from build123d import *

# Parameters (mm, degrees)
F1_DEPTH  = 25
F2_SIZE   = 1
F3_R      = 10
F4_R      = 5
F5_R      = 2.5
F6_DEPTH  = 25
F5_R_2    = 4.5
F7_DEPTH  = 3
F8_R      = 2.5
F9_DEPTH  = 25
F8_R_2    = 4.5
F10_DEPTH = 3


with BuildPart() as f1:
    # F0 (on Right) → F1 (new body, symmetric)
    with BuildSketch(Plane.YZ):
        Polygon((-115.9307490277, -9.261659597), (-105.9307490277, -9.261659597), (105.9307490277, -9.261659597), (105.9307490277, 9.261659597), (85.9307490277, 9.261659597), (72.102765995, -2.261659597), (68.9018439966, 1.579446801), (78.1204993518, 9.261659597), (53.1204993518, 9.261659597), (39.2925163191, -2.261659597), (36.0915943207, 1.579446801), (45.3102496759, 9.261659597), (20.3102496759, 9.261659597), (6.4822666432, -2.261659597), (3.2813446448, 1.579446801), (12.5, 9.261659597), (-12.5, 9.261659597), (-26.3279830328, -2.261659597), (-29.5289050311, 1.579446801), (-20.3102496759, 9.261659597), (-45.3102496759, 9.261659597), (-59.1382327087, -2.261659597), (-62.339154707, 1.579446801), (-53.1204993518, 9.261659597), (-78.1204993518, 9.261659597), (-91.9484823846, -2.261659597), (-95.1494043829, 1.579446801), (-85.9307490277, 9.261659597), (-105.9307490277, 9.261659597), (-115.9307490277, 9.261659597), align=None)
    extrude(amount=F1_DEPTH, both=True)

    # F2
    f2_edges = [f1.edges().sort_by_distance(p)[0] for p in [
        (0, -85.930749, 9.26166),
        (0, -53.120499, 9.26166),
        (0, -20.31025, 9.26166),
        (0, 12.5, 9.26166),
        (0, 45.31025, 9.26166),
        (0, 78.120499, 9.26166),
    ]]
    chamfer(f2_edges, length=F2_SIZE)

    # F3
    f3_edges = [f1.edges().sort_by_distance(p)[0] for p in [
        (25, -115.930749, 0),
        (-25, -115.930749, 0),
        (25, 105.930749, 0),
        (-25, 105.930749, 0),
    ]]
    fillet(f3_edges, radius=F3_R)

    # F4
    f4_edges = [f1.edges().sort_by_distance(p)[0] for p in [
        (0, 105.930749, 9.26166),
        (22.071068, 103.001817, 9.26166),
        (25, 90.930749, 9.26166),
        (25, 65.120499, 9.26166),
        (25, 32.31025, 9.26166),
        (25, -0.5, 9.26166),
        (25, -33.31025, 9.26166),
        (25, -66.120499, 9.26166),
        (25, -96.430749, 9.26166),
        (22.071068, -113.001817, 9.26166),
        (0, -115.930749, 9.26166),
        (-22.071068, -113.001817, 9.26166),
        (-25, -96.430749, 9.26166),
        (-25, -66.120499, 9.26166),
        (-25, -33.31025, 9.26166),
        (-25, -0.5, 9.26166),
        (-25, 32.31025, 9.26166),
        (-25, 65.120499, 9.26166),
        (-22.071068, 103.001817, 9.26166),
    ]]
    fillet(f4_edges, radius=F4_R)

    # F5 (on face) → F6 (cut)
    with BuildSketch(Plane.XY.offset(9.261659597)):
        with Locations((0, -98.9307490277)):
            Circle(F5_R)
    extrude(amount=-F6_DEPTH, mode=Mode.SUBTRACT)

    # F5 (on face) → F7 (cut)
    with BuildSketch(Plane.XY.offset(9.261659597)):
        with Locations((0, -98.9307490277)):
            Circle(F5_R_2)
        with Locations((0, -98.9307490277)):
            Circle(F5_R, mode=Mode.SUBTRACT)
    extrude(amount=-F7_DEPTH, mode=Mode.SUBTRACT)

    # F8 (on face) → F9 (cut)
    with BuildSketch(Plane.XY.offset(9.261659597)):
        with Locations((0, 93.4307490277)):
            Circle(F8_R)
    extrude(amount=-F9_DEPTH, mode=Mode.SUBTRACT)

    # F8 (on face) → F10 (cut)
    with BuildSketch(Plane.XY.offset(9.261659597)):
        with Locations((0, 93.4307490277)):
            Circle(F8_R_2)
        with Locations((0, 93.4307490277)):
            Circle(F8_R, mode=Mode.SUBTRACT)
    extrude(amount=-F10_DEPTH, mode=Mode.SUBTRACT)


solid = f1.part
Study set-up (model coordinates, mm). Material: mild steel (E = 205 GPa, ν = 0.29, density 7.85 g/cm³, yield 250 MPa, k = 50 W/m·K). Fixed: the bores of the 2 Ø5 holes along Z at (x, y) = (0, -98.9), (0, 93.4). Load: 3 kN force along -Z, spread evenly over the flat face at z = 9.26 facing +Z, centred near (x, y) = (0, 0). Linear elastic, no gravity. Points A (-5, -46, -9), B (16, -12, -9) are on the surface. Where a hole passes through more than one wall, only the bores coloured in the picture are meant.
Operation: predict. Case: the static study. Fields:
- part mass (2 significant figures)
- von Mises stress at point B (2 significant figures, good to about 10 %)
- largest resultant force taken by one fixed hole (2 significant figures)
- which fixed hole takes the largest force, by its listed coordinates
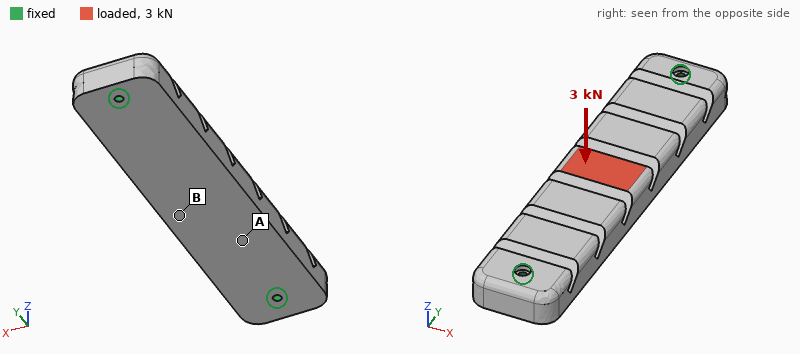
1.4 kg
31 MPa
1.7 kN
(0, 93.4)
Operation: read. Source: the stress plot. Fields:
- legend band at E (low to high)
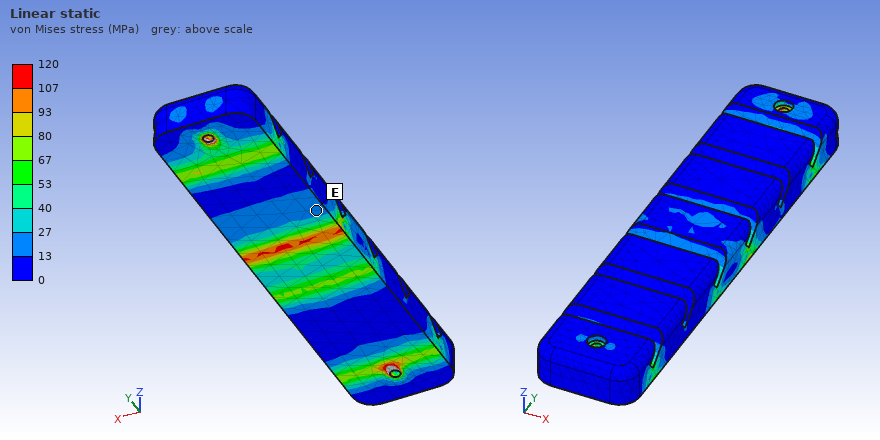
13 to 27 MPa
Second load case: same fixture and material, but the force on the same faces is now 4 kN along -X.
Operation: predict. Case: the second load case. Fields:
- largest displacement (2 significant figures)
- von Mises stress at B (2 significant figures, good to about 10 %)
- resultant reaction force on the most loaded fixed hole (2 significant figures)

41 µm
34 MPa
2.0 kN
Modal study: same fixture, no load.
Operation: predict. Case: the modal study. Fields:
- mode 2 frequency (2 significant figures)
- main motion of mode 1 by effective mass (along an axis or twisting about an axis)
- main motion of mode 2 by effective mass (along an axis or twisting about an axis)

2500 Hz
along Z
along X
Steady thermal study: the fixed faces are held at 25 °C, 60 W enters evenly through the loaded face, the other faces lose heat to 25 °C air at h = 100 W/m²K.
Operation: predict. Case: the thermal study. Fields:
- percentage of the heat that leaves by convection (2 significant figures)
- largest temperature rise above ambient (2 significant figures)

83 %
65 K
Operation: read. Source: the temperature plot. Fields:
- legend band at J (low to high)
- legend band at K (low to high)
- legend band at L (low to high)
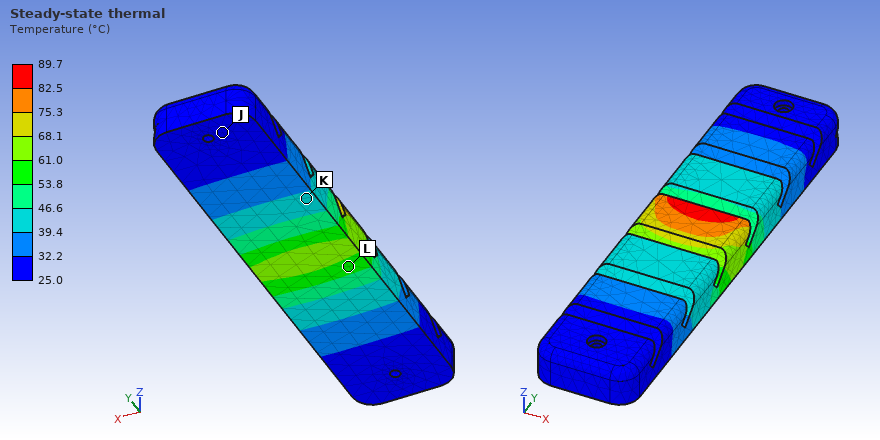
25.0 to 32.2 °C
39.4 to 46.6 °C
53.8 to 61.0 °C
